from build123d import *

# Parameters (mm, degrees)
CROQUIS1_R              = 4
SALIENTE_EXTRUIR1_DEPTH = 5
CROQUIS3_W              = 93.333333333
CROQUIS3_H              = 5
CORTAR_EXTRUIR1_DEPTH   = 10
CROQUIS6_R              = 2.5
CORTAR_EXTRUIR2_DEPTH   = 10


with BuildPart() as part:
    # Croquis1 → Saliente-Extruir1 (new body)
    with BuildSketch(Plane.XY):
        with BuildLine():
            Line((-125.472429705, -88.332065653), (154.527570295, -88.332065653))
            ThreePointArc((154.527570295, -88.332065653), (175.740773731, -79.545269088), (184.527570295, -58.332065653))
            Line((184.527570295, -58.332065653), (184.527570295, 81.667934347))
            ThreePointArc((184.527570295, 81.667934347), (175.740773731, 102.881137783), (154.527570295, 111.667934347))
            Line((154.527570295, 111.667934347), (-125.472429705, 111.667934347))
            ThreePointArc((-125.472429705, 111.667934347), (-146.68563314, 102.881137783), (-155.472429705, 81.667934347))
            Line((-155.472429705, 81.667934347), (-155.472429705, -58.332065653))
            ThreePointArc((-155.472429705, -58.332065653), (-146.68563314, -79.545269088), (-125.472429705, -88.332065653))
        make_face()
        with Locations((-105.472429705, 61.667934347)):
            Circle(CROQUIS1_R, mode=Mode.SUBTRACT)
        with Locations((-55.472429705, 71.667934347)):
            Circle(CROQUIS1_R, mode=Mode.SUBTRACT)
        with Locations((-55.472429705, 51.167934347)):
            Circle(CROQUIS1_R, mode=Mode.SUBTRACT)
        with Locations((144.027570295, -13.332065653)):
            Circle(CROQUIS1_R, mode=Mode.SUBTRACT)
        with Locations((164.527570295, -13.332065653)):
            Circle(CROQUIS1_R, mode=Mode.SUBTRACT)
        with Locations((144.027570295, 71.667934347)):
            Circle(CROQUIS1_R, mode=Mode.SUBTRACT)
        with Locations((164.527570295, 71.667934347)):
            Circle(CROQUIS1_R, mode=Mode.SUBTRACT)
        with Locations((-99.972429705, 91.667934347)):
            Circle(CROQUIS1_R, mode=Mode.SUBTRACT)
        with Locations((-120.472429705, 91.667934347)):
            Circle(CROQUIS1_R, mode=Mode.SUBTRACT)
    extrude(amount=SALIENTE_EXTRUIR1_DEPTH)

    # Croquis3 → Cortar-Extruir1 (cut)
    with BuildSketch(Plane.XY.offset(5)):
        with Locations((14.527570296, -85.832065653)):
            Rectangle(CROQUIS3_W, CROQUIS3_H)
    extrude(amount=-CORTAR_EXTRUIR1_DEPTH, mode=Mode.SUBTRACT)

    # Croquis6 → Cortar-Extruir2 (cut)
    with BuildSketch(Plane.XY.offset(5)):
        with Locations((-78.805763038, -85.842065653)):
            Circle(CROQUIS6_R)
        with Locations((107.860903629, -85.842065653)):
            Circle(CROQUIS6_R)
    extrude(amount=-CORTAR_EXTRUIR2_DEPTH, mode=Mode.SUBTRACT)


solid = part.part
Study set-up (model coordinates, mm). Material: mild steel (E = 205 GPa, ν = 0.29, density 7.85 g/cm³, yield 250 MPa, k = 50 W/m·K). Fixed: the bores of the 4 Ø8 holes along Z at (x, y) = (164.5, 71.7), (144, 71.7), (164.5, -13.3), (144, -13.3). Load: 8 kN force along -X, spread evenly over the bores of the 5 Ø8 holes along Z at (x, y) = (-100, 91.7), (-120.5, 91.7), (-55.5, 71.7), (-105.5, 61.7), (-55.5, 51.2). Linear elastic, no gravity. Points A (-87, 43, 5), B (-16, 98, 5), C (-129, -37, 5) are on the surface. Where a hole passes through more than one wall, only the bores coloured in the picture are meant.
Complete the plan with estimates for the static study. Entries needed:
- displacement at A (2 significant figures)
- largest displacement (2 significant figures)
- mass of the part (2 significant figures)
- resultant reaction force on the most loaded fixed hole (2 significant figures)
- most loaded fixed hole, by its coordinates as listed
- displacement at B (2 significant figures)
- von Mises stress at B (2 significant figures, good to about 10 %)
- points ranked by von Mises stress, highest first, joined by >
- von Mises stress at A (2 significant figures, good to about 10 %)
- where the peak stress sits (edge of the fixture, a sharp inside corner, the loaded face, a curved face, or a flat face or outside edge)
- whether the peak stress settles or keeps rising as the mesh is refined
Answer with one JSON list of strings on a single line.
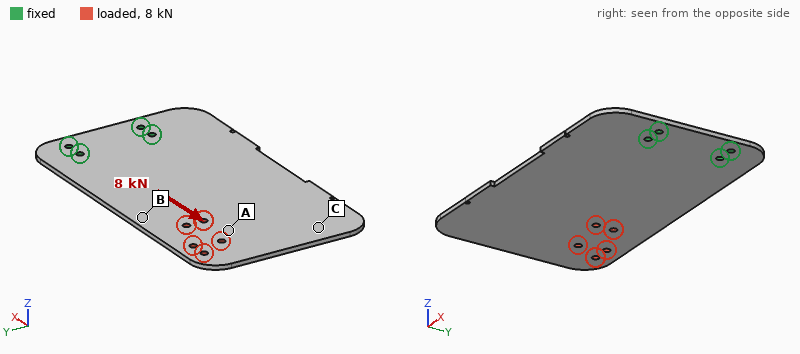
["33 µm", "52 µm", "2.6 kg", "5.3 kN", "(144, 71.7)", "27 µm", "20 MPa", "B > A > C", "6.9 MPa", "edge of the fixture", "keeps rising"]
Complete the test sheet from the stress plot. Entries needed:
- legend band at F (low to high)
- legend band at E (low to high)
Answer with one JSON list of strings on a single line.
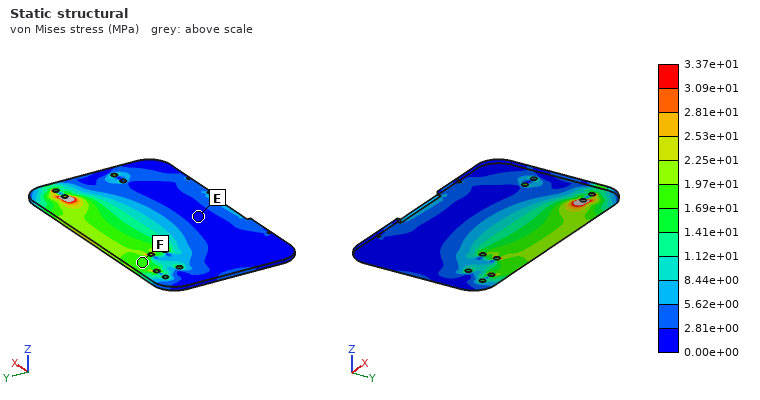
["1.69e+01 to 1.97e+01 MPa", "0.00e+00 to 2.81e+00 MPa"]
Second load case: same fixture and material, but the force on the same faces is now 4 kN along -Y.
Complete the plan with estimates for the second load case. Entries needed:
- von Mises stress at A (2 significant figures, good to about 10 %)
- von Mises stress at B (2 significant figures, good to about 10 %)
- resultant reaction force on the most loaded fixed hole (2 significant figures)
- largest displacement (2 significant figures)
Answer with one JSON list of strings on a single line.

["7.4 MPa", "8.9 MPa", "7.5 kN", "97 µm"]
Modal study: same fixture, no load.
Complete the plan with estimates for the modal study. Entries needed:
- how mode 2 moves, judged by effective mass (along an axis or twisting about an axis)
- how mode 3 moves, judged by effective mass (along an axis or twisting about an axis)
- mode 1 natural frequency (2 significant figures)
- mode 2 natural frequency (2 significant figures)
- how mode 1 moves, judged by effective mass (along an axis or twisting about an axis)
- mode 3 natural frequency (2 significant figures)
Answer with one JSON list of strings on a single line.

["twisting about X", "along Z", "46 Hz", "150 Hz", "along Z", "280 Hz"]
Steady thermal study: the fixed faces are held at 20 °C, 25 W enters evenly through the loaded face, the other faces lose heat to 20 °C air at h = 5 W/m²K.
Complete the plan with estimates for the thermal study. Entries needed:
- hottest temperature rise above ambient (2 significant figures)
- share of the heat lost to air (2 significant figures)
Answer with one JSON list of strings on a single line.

["77 K", "72 %"]
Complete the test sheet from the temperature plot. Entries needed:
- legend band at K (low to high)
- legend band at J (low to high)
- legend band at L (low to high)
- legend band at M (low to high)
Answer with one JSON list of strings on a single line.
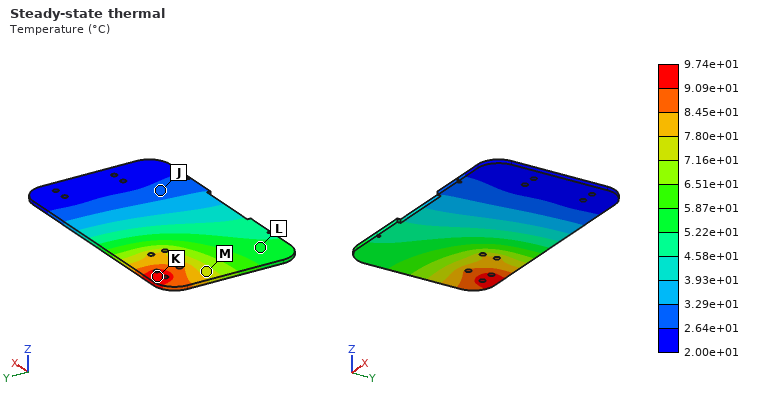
["9.09e+01 to 9.74e+01 °C", "2.64e+01 to 3.29e+01 °C", "5.22e+01 to 5.87e+01 °C", "7.16e+01 to 7.80e+01 °C"]
